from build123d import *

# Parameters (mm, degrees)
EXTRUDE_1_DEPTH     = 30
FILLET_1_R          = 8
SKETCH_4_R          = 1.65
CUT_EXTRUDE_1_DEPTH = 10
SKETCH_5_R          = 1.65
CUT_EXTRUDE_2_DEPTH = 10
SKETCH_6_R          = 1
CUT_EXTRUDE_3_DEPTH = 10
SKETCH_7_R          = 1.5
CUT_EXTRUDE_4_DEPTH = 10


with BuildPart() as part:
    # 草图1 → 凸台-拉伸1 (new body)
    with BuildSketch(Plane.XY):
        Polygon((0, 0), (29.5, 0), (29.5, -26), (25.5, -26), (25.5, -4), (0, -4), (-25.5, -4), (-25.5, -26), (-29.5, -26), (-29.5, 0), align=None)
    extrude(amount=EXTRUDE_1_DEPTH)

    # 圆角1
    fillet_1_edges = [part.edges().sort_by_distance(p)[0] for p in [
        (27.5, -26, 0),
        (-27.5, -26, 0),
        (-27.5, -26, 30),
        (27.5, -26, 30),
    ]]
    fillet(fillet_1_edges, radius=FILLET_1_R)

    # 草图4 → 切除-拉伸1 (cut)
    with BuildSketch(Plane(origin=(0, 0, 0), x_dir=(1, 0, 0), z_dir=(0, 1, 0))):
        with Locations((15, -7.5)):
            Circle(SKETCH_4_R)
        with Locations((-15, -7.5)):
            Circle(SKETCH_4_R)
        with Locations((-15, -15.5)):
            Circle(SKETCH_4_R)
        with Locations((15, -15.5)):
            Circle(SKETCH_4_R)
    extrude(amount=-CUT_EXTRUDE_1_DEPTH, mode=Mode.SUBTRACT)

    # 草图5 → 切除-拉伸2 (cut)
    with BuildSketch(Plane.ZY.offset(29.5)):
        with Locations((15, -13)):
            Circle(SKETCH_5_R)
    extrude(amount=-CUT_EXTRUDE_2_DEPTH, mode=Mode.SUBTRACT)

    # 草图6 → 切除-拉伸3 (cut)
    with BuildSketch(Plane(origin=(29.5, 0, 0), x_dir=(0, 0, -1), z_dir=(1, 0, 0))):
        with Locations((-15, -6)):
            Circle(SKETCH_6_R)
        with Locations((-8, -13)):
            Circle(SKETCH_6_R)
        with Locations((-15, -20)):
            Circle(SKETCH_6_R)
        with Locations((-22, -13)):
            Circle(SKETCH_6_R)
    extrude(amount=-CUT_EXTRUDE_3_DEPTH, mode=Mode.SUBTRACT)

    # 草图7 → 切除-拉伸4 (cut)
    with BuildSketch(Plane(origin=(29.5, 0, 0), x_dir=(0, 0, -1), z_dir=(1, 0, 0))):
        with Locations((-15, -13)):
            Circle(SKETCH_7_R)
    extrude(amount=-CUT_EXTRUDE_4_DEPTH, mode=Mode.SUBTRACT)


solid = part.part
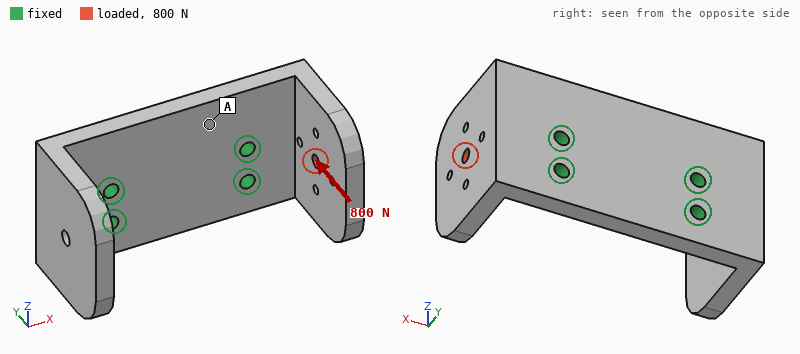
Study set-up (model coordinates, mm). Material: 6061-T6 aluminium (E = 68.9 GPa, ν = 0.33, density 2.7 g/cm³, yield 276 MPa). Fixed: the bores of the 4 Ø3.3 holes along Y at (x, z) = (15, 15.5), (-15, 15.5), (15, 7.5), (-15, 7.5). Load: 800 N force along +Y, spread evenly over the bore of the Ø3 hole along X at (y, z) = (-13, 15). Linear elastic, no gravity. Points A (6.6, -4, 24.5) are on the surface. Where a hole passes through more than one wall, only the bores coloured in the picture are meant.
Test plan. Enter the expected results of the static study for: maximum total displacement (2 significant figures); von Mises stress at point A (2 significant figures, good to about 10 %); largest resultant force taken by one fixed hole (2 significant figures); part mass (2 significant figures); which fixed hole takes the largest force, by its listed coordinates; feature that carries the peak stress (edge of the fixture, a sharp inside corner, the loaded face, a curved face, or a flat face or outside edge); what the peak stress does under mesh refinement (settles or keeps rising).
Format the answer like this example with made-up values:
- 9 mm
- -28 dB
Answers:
- 0.16 mm
- 20 MPa
- 640 N
- 32 g
- (15, 15.5)
- edge of the fixture
- keeps rising
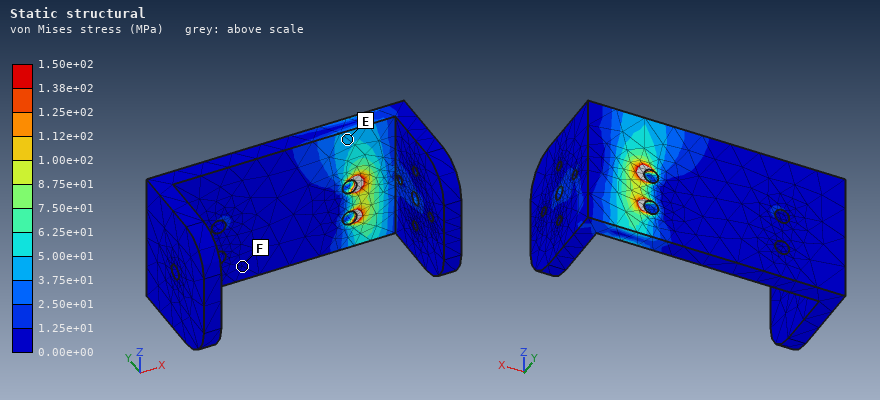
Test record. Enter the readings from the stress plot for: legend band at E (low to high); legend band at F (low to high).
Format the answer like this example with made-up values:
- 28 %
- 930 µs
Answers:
- 3.75e+01 to 5.00e+01 MPa
- 0.00e+00 to 1.25e+01 MPa
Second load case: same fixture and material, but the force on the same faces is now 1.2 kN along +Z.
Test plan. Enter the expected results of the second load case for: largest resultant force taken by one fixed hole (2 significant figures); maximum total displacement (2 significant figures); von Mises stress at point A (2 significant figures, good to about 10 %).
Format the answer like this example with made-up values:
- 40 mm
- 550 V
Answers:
- 1.3 kN
- 0.17 mm
- 28 MPa
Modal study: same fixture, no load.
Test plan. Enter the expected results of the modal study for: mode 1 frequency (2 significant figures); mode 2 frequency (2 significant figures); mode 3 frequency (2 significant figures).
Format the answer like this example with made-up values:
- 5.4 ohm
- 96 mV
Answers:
- 3300 Hz
- 3300 Hz
- 5100 Hz
